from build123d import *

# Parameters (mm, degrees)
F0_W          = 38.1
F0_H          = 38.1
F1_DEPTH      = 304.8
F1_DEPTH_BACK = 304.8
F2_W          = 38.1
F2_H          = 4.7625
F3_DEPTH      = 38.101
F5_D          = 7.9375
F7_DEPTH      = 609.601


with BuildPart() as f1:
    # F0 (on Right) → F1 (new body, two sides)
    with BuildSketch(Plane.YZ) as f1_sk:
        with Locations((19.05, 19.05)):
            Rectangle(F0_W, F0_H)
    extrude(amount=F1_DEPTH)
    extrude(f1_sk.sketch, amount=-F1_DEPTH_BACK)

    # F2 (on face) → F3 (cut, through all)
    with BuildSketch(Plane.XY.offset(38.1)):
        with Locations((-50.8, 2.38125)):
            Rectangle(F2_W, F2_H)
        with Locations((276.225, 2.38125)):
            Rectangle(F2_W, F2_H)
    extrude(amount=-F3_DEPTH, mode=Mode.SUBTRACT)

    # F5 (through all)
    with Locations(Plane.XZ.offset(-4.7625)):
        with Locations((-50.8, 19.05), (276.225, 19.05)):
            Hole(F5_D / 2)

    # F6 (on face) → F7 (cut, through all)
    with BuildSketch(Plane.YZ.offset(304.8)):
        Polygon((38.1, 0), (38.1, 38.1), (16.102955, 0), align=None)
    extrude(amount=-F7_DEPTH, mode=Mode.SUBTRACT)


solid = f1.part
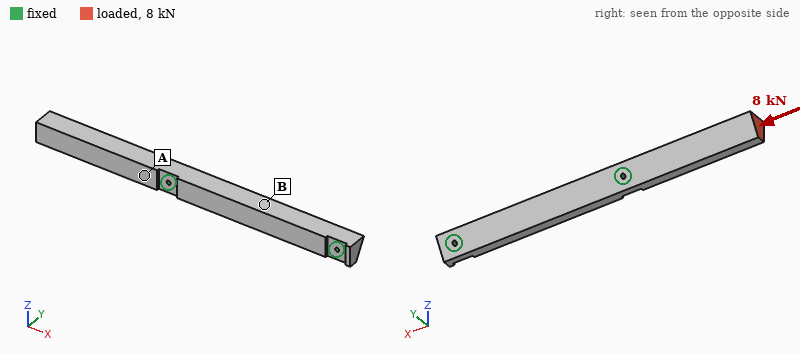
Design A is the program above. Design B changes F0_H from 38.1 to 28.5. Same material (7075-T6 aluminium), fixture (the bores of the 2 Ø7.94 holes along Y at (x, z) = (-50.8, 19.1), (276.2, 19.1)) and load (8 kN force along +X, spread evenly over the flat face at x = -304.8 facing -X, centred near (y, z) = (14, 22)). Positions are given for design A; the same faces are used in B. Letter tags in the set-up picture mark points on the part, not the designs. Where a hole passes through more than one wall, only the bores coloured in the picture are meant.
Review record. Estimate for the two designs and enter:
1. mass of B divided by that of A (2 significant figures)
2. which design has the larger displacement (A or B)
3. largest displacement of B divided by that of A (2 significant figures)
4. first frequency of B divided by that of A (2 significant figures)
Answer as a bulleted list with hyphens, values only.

- 0.75
- B
- 1.2
- 0.93
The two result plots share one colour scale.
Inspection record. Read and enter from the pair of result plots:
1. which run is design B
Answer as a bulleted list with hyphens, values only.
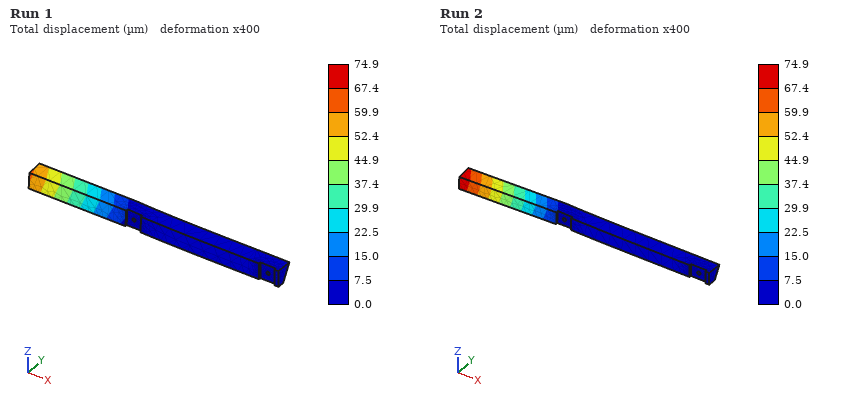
- Run 2
